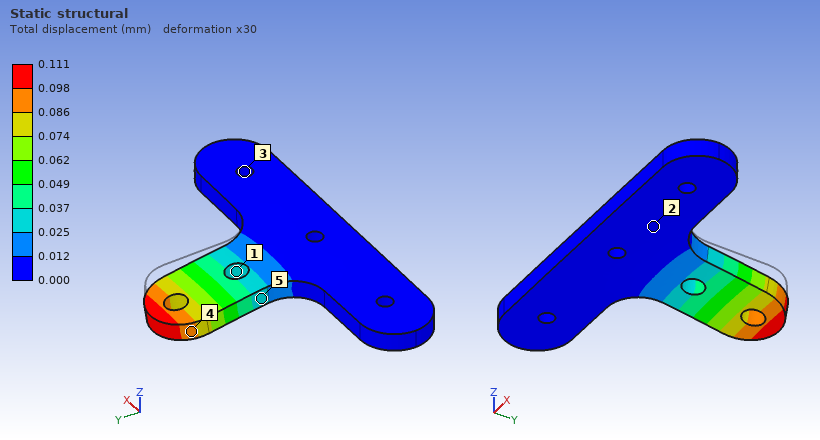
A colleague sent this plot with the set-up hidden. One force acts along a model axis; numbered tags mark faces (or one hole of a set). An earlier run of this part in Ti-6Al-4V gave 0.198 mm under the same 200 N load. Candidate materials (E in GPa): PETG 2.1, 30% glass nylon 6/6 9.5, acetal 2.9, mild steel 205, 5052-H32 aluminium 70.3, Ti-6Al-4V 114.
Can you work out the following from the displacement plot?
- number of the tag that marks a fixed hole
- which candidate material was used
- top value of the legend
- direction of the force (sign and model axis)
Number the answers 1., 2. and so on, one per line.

1. 3
2. mild steel
3. 0.111 mm
4. -Z
